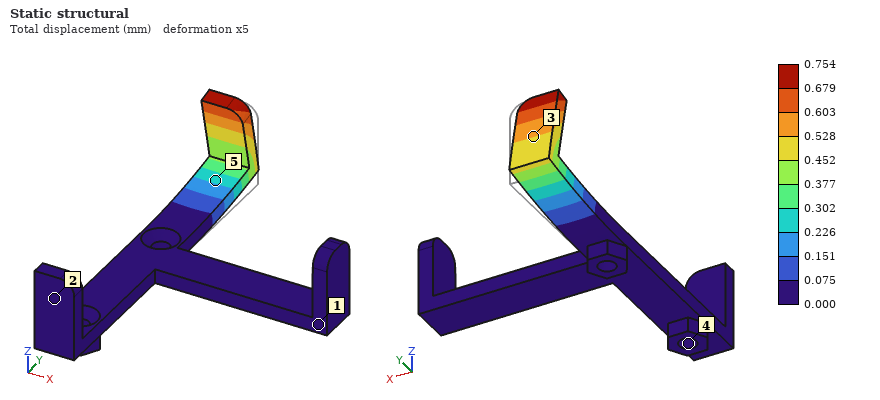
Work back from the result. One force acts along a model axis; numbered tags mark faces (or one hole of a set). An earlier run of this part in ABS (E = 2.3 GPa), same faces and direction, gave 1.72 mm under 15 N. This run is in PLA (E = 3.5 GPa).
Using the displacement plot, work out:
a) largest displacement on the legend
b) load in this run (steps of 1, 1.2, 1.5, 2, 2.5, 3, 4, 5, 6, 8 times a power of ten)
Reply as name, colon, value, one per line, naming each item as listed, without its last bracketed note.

largest displacement on the legend: 0.754 mm
load in this run: 10 N
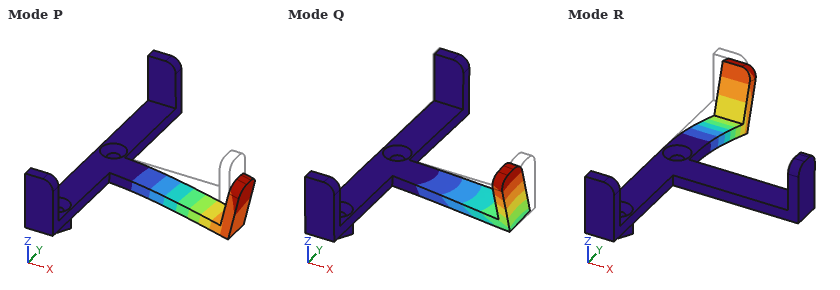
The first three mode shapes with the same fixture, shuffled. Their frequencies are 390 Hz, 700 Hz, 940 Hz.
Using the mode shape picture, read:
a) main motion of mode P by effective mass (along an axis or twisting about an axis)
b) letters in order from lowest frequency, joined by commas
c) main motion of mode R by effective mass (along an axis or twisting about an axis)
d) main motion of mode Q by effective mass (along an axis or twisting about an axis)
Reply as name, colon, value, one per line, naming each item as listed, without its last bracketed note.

main motion of mode P by effective mass: along Z
letters in order from lowest frequency, joined by commas: P, R, Q
main motion of mode R by effective mass: along Z
main motion of mode Q by effective mass: along Y
